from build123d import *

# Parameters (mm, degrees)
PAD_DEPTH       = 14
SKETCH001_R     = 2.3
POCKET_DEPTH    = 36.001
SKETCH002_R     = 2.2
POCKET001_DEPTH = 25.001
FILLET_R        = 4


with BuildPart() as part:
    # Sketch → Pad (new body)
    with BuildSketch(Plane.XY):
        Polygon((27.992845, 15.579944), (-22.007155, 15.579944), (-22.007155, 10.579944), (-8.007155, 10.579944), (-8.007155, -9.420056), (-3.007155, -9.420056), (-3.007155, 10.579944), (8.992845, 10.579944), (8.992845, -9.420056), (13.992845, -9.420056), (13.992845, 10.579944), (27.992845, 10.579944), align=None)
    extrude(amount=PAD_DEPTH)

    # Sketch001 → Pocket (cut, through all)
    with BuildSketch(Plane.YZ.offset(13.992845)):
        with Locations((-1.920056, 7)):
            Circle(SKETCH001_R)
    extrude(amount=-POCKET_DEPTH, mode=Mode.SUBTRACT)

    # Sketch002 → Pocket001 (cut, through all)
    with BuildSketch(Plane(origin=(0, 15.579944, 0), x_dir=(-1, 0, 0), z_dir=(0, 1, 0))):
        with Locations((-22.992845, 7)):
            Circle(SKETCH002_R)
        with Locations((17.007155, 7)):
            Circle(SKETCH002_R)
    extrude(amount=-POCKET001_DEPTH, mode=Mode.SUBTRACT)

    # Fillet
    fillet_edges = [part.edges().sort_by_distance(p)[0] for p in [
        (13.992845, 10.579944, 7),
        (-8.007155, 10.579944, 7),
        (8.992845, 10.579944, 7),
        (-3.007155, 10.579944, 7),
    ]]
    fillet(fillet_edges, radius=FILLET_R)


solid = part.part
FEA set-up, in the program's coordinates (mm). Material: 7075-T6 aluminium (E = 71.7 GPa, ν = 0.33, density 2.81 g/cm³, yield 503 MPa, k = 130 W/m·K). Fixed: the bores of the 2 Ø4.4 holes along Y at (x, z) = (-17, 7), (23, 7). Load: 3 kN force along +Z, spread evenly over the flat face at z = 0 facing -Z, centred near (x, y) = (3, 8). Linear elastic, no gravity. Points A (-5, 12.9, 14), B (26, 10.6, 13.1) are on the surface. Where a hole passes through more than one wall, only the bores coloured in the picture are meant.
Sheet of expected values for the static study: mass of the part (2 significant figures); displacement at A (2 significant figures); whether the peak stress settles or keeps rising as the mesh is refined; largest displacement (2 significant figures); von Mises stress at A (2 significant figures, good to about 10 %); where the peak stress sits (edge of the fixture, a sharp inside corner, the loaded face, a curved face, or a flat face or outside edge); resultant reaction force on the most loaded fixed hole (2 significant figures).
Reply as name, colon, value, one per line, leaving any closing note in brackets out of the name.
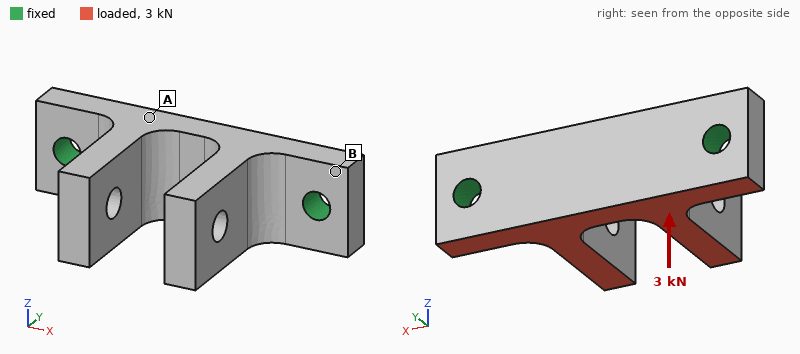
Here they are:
mass of the part: 17 g
displacement at A: 0.034 mm
whether the peak stress settles or keeps rising as the mesh is refined: keeps rising
largest displacement: 0.13 mm
von Mises stress at A: 37 MPa
where the peak stress sits: edge of the fixture
resultant reaction force on the most loaded fixed hole: 1.5 kN
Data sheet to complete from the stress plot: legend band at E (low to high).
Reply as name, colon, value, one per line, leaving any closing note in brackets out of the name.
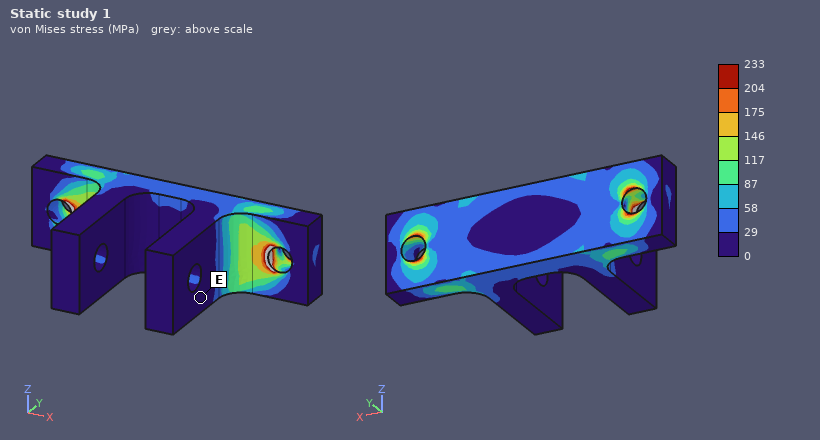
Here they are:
legend band at E: 0 to 29 MPa
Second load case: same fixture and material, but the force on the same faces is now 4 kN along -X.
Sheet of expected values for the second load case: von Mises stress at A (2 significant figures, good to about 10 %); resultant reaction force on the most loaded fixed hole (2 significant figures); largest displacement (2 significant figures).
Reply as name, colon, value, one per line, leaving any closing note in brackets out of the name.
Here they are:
von Mises stress at A: 33 MPa
resultant reaction force on the most loaded fixed hole: 2.2 kN
largest displacement: 0.12 mm
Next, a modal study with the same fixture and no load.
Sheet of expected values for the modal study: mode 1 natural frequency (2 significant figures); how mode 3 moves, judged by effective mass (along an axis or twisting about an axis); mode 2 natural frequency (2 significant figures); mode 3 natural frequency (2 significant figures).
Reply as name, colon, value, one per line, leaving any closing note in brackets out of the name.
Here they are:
mode 1 natural frequency: 7000 Hz
how mode 3 moves, judged by effective mass: along X
mode 2 natural frequency: 7100 Hz
mode 3 natural frequency: 10 kHz
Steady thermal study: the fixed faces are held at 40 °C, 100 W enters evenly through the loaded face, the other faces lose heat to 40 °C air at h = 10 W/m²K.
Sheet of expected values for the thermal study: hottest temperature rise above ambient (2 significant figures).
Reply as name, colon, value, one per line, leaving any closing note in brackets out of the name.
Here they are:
hottest temperature rise above ambient: 74 K
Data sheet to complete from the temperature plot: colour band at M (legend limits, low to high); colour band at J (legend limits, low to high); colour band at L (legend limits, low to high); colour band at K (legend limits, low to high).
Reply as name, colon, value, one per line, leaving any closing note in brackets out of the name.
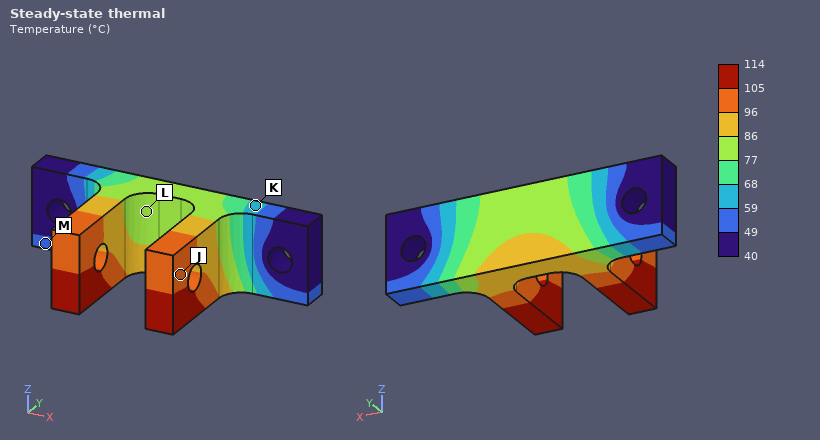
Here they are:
colour band at M: 49 to 59 °C
colour band at J: 96 to 105 °C
colour band at L: 77 to 86 °C
colour band at K: 59 to 68 °C
